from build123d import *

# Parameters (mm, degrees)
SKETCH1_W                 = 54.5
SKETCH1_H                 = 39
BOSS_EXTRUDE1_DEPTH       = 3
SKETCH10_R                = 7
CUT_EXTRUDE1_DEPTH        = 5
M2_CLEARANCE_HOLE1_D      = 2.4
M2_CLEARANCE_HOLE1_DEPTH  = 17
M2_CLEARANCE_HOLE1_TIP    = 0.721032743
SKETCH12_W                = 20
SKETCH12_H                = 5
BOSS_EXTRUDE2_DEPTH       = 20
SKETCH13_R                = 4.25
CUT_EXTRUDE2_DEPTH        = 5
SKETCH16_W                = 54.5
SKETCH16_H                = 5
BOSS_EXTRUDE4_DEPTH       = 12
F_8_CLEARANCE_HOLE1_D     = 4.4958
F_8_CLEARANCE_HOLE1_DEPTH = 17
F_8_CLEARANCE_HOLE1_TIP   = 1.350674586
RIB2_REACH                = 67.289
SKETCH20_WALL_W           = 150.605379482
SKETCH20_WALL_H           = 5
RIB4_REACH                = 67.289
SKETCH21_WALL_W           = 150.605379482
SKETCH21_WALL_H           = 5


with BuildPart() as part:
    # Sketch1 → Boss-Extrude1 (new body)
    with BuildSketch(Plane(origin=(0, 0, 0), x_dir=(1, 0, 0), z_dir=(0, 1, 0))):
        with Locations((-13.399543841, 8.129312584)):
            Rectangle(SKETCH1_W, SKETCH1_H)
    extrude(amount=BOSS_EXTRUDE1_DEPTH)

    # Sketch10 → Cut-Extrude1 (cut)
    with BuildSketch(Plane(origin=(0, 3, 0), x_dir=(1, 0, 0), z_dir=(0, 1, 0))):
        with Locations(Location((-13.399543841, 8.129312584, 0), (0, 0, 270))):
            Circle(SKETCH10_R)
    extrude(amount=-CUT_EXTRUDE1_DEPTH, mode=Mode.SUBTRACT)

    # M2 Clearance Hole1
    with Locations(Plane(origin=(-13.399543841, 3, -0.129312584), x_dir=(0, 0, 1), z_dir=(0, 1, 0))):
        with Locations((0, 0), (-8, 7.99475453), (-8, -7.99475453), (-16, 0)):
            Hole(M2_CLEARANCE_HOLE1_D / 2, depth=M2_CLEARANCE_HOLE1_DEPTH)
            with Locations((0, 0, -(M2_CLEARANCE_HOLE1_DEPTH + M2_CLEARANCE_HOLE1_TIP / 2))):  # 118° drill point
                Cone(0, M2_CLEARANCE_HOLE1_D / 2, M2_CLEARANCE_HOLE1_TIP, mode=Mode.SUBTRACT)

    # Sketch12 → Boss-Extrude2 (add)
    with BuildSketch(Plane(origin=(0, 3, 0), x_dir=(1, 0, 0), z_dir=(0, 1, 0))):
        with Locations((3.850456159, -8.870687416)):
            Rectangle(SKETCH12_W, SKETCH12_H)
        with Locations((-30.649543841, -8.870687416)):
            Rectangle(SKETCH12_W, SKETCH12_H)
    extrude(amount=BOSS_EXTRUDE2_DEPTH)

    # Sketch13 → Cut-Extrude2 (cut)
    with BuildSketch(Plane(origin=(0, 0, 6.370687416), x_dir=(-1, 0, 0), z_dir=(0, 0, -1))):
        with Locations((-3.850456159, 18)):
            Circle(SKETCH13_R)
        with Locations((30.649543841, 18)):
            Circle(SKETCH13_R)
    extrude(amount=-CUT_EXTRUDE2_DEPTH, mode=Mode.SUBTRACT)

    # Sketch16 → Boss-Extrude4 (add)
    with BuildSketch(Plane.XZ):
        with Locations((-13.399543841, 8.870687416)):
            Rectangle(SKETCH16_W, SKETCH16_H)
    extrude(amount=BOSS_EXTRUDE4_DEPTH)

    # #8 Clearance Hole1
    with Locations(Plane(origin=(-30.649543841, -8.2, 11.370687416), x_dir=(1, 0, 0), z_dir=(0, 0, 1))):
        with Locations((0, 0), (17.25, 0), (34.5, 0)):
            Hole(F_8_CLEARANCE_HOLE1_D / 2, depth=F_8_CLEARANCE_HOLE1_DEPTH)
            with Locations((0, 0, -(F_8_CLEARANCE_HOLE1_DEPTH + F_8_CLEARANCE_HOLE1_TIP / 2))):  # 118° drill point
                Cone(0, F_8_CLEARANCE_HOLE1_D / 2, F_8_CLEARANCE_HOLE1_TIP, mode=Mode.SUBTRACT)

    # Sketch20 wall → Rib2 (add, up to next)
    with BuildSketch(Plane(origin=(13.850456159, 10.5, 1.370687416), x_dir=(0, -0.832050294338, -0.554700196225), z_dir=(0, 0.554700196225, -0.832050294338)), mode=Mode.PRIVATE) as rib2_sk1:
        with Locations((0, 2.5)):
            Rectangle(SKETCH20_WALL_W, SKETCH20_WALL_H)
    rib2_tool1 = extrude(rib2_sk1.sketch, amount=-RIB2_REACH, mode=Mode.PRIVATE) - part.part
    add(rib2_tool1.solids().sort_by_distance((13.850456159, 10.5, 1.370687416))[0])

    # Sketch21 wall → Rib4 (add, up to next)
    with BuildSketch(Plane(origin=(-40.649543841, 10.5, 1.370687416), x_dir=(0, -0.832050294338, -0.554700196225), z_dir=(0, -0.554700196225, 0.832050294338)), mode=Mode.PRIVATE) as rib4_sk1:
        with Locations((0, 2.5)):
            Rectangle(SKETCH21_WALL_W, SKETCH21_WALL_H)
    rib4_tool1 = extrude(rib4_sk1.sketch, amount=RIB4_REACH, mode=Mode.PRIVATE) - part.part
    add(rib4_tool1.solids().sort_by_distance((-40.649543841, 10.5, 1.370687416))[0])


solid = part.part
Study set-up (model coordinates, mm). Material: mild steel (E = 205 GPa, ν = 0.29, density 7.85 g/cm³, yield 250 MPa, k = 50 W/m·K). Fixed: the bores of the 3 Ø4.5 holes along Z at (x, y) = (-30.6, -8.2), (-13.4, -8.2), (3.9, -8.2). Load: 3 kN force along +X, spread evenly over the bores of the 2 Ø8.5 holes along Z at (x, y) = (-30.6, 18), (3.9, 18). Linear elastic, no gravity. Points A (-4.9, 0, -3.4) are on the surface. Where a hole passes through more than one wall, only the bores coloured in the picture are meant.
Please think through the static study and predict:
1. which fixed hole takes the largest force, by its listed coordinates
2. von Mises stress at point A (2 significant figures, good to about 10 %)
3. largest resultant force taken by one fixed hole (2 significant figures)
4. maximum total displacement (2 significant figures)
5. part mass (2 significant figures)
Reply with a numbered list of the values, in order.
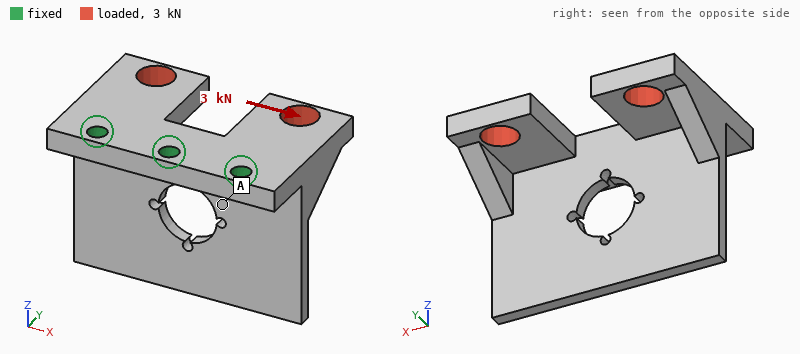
1. (-13.4, -8.2)
2. 14 MPa
3. 2.5 kN
4. 28 µm
5. 100 g
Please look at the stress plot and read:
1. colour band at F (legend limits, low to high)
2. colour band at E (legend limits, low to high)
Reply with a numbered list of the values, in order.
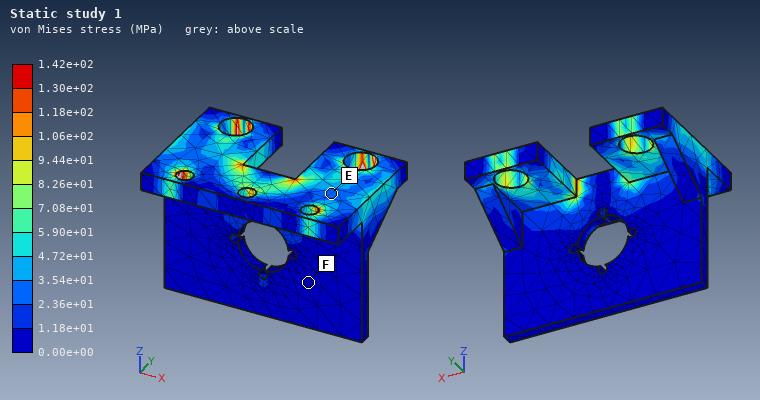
1. 0.00e+00 to 1.18e+01 MPa
2. 2.36e+01 to 3.54e+01 MPa
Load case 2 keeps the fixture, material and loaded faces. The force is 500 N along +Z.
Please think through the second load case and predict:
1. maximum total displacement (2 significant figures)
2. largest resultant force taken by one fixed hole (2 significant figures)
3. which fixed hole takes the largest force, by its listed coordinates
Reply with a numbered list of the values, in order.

1. 40 µm
2. 230 N
3. (-13.4, -8.2)
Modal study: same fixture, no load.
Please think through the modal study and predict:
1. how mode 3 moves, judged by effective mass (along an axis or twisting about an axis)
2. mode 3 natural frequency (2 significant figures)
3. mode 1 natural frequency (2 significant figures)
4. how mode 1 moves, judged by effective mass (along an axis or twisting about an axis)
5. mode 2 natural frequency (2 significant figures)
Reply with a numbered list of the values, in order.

1. along Z
2. 5600 Hz
3. 2000 Hz
4. along Y
5. 3500 Hz
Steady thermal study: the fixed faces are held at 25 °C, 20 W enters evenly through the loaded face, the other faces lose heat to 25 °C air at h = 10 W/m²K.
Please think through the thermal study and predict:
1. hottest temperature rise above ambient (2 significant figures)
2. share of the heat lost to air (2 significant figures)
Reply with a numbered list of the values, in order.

1. 59 K
2. 7.2 %
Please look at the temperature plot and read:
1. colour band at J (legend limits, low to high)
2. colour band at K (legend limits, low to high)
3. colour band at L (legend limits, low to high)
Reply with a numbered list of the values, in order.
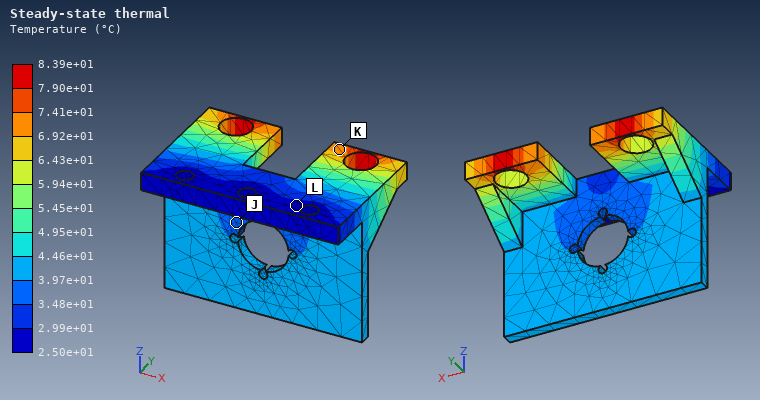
1. 3.48e+01 to 3.97e+01 °C
2. 6.92e+01 to 7.41e+01 °C
3. 2.50e+01 to 2.99e+01 °C
